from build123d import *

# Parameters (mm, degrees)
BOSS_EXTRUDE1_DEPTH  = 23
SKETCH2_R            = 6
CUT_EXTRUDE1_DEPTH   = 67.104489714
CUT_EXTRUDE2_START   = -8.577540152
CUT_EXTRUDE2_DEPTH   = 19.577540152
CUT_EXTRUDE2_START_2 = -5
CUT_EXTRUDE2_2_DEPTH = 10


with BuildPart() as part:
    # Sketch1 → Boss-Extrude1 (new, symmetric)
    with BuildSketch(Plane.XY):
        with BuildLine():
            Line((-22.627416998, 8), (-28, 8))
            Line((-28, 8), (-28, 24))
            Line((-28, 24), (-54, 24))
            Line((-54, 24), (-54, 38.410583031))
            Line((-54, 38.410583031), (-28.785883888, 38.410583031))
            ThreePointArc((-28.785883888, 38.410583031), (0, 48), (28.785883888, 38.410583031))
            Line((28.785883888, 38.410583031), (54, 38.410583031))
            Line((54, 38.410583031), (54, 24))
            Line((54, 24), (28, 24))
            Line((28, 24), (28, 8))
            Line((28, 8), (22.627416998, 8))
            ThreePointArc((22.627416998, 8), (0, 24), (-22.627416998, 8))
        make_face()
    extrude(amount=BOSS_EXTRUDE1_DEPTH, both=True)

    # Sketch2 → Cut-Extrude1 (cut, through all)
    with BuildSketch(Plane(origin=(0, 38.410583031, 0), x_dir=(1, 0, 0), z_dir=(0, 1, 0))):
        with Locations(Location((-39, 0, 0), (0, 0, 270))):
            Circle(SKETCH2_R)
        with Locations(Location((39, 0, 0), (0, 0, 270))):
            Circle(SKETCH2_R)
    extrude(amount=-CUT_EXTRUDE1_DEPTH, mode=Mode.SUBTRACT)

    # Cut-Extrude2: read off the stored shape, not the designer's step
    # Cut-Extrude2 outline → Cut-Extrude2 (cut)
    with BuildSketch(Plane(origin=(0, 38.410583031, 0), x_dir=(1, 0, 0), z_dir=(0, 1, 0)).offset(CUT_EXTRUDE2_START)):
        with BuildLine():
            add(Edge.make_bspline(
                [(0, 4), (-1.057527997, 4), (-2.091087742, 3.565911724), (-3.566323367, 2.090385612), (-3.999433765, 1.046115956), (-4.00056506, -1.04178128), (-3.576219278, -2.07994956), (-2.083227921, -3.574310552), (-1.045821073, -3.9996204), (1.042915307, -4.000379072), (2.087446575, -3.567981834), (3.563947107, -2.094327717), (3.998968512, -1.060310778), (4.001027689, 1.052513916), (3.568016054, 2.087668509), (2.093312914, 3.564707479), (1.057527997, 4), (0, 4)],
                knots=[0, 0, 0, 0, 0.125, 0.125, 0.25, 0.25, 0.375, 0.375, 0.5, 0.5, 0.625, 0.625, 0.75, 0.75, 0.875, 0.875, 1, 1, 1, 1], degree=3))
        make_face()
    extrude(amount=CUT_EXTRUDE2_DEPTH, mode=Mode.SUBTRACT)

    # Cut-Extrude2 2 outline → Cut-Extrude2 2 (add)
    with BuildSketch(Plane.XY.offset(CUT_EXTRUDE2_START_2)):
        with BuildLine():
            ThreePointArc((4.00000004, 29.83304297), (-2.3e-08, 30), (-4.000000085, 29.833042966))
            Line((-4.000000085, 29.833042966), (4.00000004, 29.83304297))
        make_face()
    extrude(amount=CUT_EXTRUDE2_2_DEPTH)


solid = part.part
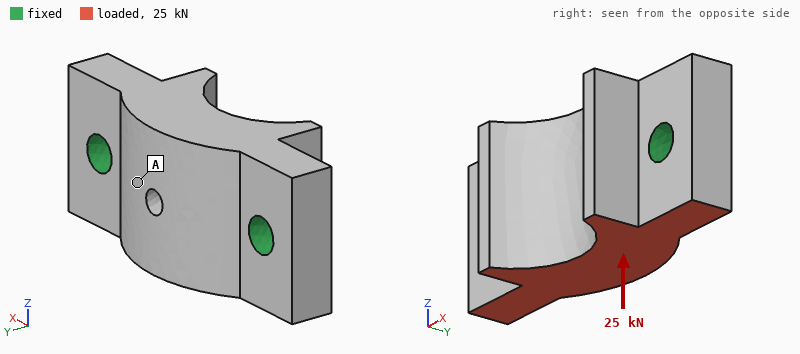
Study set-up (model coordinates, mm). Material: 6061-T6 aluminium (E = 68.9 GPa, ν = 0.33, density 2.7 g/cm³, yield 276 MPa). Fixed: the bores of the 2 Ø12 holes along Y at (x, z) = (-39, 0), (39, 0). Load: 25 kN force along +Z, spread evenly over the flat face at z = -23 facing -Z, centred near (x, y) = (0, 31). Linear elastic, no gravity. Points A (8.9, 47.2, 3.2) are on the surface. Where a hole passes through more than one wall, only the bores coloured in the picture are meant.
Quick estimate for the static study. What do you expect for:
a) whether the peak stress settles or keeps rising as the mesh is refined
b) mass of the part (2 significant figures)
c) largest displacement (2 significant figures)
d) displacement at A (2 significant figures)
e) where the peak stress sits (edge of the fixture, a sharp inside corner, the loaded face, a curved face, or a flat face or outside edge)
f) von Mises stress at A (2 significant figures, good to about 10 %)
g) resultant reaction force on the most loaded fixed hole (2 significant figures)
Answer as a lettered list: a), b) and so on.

a) keeps rising
b) 270 g
c) 20 µm
d) 16 µm
e) edge of the fixture
f) 9.9 MPa
g) 13 kN
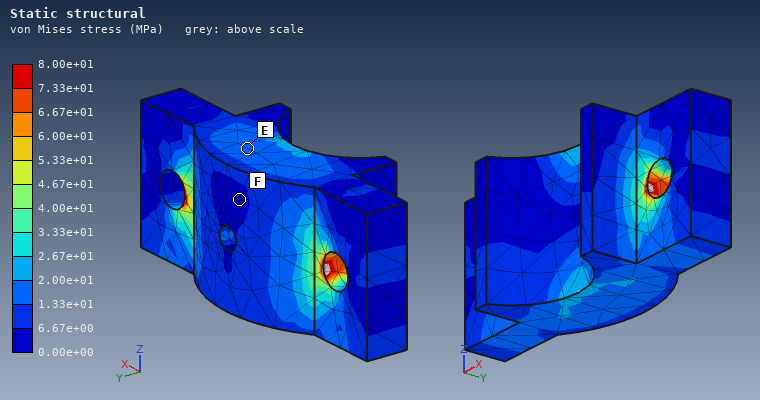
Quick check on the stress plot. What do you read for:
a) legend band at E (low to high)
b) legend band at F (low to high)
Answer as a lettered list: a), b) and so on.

a) 1.33e+01 to 2.00e+01 MPa
b) 0.00e+00 to 6.67e+00 MPa
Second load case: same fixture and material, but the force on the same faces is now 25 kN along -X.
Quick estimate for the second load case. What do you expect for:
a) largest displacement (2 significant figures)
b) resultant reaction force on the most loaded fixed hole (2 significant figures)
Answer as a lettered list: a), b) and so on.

a) 29 µm
b) 14 kN
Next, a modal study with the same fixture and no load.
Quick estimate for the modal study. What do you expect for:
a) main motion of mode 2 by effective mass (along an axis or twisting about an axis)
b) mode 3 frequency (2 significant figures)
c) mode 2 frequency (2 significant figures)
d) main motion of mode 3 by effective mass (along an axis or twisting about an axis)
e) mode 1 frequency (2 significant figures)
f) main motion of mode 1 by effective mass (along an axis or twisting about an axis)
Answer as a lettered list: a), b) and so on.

a) along Y
b) 12 kHz
c) 10000 Hz
d) along Z
e) 8700 Hz
f) twisting about X
